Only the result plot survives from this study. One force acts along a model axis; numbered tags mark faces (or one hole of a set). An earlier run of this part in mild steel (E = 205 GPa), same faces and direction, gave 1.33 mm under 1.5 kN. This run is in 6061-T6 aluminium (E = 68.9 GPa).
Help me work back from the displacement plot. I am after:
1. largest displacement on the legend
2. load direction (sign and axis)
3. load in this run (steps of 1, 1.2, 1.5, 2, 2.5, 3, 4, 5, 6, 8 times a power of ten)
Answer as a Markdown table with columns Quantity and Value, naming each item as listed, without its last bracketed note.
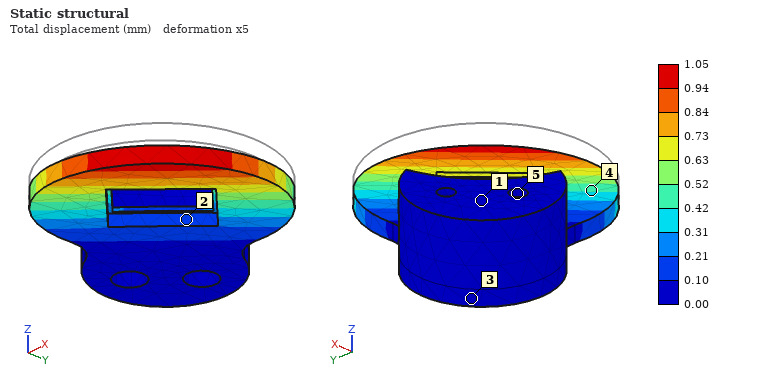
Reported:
| Quantity | Value |
|---|---|
| largest displacement on the legend | 1.05 mm |
| load direction | -Z |
| load in this run | 400 N |
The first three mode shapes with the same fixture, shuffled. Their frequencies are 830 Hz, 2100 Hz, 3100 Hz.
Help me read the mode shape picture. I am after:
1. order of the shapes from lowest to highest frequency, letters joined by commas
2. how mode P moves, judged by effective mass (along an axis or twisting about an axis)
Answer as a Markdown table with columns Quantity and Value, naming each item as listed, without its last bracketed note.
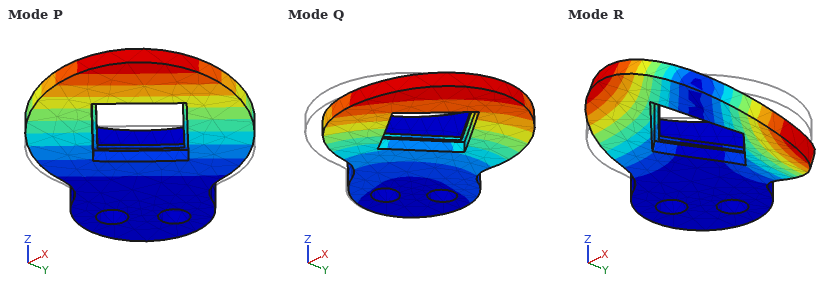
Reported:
| Quantity | Value |
|---|---|
| order of the shapes from lowest to highest frequency, letters joined by commas | P, R, Q |
| how mode P moves, judged by effective mass | along Z |
